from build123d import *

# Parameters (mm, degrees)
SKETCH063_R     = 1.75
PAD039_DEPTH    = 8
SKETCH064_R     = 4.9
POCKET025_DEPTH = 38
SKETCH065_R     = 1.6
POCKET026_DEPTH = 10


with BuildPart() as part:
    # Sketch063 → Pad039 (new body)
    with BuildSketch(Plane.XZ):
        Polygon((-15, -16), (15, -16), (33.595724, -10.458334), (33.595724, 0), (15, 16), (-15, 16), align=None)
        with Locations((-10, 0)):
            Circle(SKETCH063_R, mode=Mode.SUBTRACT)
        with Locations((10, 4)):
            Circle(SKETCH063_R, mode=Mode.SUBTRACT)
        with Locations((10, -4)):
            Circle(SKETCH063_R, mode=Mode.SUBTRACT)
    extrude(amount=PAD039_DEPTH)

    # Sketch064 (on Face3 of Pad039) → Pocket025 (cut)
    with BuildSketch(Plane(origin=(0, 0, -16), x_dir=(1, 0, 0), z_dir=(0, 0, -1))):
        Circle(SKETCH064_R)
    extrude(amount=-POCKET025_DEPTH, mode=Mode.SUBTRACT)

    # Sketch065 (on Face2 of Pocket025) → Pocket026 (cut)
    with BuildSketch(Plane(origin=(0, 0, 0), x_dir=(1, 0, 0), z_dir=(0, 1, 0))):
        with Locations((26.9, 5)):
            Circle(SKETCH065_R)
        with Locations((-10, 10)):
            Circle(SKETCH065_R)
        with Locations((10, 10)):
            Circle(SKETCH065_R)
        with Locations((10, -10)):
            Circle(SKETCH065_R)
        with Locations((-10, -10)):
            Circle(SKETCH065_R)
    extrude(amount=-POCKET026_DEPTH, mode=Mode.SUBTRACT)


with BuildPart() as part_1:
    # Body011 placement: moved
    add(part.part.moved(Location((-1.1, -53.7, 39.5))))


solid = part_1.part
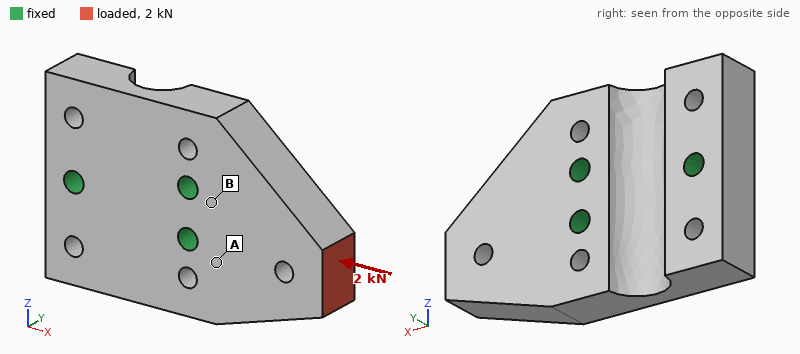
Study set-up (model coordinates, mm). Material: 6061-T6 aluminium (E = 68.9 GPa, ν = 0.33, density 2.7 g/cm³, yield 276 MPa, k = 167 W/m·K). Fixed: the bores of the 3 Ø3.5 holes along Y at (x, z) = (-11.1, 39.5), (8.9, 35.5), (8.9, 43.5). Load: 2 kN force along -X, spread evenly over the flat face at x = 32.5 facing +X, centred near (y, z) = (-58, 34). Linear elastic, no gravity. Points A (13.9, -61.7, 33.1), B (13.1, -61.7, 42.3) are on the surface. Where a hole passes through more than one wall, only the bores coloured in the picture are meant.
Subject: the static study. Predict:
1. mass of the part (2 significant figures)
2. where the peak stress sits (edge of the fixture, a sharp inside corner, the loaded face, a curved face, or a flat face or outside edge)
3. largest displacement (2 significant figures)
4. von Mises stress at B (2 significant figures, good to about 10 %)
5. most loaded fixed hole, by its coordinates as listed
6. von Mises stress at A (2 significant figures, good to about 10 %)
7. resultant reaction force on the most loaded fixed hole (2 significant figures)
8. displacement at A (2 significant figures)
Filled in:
25 g
a curved face
9.4 µm
6.7 MPa
(8.9, 35.5)
20 MPa
1.6 kN
2.1 µm
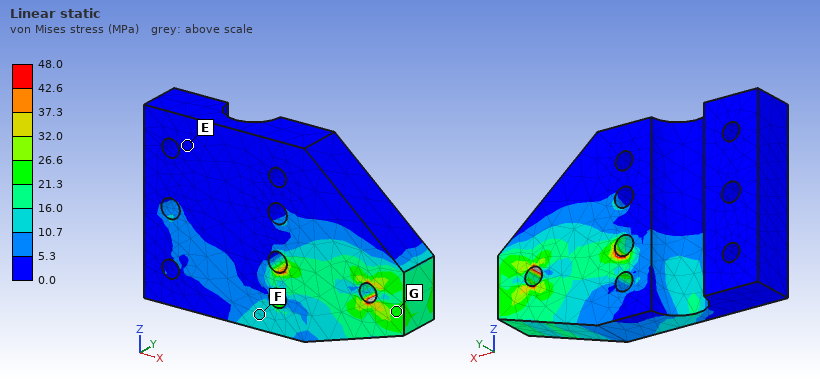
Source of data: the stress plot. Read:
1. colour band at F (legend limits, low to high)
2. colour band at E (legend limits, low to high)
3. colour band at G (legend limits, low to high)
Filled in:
10.7 to 16.0 MPa
0.0 to 5.3 MPa
21.3 to 26.6 MPa
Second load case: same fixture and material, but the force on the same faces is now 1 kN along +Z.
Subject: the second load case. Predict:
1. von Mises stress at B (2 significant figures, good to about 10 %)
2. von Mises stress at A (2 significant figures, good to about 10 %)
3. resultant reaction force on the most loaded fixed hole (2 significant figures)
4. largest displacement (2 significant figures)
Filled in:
25 MPa
15 MPa
1.5 kN
19 µm
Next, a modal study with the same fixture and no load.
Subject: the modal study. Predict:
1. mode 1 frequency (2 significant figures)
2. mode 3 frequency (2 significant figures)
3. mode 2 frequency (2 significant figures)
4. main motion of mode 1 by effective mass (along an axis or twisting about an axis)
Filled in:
13 kHz
23 kHz
22 kHz
along Y
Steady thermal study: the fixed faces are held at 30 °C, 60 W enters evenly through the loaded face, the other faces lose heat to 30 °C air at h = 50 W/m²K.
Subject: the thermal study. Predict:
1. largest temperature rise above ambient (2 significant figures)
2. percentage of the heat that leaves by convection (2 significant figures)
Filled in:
62 K
3.1 %
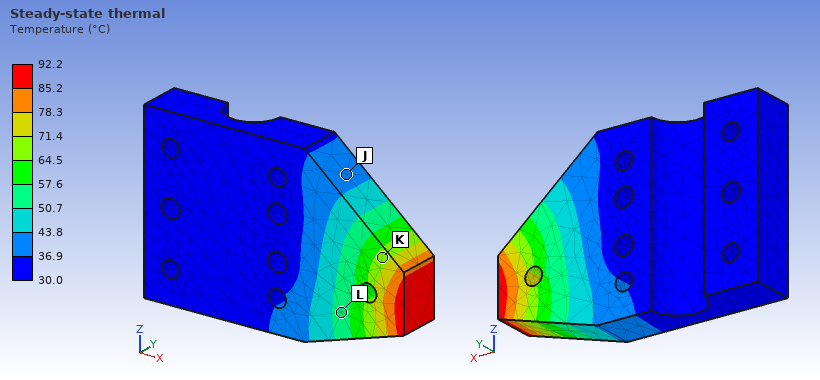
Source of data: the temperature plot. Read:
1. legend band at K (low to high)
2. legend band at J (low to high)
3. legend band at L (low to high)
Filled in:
64.5 to 71.4 °C
36.9 to 43.8 °C
50.7 to 57.6 °C
